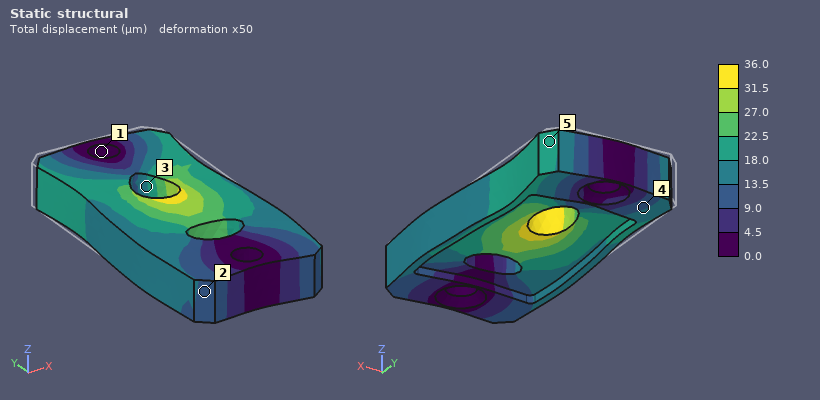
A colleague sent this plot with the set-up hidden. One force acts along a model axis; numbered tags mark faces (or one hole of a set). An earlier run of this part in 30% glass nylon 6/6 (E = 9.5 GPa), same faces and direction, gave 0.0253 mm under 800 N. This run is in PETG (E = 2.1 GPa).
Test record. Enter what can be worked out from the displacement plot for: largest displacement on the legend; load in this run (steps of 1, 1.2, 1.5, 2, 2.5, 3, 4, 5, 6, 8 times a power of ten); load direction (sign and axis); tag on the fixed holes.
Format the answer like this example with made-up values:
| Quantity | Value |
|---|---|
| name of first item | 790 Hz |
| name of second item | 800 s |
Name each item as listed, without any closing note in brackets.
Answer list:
| Quantity | Value |
|---|---|
| largest displacement on the legend | 36.0 µm |
| load in this run | 250 N |
| load direction | -Y |
| tag on the fixed holes | 1 |
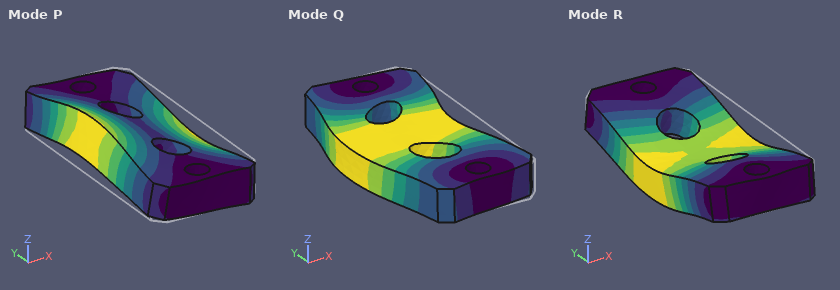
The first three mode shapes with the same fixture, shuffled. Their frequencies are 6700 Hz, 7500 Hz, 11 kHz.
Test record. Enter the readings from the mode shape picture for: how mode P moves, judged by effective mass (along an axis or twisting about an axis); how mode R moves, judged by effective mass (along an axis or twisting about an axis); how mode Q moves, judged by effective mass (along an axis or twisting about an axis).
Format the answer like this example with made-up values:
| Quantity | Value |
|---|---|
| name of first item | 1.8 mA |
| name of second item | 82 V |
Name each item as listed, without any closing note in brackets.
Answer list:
| Quantity | Value |
|---|---|
| how mode P moves, judged by effective mass | twisting about Y |
| how mode R moves, judged by effective mass | along Z |
| how mode Q moves, judged by effective mass | along X |
